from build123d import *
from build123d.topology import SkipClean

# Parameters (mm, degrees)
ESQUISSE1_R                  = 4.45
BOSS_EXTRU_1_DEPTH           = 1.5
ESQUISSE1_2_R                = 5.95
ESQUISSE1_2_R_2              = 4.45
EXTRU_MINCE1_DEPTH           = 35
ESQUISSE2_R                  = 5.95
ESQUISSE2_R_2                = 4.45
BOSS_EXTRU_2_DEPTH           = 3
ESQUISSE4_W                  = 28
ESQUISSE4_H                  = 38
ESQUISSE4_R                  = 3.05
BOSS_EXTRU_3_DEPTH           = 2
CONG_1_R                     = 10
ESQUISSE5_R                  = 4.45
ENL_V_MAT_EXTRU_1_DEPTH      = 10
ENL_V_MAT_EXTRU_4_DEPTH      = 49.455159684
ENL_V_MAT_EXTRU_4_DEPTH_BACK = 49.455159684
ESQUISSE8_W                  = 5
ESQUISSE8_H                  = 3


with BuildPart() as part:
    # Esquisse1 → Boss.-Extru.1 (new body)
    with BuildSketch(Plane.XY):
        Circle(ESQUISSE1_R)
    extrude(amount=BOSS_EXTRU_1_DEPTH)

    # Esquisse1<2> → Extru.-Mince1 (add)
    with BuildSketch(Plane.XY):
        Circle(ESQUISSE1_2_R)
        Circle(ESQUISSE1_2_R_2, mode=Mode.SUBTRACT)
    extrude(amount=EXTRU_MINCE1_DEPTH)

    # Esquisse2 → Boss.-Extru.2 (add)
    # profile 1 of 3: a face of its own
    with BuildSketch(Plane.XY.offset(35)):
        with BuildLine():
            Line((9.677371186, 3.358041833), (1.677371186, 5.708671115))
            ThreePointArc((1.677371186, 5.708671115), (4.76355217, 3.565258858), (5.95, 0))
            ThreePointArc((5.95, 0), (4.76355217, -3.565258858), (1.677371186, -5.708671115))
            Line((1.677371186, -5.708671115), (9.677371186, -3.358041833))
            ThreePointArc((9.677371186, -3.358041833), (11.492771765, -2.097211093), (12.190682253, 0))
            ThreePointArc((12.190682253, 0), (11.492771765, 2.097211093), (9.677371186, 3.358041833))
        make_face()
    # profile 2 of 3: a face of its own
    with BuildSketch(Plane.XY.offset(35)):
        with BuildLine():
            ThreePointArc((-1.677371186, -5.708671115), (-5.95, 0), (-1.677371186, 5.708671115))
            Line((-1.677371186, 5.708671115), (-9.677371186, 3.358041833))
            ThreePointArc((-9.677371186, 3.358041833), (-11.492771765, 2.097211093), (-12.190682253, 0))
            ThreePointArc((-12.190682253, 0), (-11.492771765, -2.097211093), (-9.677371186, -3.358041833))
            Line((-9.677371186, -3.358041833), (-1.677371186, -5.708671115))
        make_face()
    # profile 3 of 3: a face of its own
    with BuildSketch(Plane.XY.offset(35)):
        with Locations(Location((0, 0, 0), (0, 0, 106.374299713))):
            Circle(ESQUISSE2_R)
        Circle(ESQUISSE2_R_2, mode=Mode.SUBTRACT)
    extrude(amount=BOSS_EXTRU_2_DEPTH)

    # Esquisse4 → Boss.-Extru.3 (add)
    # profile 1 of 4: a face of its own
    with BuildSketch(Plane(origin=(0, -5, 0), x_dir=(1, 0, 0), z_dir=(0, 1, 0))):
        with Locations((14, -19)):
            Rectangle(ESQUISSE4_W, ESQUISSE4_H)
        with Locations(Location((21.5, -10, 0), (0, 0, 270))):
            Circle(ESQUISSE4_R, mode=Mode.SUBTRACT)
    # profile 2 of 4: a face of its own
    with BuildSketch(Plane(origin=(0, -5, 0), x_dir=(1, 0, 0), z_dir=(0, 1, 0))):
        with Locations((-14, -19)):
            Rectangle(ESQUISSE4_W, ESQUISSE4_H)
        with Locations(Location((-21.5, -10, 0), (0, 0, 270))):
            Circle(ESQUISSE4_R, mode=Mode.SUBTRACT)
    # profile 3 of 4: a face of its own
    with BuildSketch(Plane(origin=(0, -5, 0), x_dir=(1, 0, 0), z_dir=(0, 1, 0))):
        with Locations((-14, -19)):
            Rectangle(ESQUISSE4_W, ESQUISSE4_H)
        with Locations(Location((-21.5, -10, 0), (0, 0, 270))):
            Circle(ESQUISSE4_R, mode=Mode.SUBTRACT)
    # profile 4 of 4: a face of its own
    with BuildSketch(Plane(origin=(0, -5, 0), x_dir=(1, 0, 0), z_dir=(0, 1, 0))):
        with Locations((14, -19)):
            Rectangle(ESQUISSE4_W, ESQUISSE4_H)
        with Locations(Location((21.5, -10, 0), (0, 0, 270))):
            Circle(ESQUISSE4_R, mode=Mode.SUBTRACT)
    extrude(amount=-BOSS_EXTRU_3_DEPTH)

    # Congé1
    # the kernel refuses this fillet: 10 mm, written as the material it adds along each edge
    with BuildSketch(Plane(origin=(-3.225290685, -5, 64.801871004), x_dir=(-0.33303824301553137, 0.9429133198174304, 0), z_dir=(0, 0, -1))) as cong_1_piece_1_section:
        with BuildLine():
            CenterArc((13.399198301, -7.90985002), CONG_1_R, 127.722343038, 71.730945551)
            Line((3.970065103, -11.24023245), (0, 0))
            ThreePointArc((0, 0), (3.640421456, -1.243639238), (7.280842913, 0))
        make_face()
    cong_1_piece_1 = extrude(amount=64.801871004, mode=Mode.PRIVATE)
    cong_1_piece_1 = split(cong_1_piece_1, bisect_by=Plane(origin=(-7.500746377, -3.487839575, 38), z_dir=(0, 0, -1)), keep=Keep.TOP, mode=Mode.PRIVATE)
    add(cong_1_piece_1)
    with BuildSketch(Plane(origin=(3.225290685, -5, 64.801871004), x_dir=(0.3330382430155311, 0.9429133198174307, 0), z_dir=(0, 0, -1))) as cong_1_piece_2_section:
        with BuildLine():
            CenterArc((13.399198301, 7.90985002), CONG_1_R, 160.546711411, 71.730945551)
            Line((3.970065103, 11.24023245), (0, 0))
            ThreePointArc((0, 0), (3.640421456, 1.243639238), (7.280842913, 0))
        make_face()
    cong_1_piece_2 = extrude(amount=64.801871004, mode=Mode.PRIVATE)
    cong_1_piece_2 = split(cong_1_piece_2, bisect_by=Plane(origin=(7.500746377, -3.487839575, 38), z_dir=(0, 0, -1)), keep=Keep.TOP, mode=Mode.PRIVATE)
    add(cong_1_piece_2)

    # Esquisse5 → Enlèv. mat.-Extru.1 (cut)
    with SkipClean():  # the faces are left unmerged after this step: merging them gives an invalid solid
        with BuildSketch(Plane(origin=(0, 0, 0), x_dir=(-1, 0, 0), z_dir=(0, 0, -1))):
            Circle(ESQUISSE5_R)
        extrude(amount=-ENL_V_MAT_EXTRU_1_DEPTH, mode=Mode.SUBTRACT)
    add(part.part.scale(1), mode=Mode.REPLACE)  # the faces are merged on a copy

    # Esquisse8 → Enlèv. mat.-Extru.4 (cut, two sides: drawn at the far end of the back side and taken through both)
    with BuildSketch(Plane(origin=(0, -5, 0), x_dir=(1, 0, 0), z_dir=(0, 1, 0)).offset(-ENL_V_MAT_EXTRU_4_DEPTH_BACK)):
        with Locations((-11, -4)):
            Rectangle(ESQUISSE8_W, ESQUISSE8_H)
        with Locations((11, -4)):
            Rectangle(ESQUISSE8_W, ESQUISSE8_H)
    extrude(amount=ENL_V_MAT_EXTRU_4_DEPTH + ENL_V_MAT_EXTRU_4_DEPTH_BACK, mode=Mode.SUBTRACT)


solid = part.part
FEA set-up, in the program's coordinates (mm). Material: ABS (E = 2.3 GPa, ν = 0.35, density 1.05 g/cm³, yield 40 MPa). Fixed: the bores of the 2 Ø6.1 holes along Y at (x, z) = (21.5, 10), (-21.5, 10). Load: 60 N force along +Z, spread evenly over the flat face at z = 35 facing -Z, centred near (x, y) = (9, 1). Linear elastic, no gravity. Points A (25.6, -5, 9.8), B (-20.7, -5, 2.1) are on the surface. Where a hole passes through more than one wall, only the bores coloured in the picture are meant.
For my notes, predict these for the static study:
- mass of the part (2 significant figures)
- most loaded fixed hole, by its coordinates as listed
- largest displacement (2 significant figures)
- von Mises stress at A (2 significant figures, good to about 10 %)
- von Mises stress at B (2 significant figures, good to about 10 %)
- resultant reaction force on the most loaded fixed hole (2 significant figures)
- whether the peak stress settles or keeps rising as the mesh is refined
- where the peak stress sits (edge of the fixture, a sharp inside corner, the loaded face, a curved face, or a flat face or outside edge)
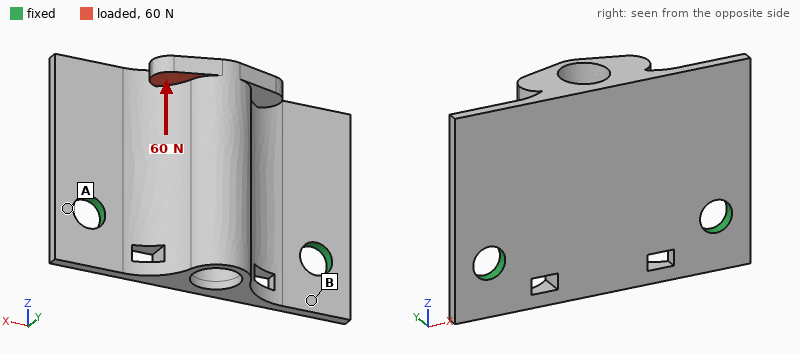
7.8 g
(21.5, 10)
0.62 mm
1.7 MPa
4.5 MPa
44 N
keeps rising
a sharp inside corner
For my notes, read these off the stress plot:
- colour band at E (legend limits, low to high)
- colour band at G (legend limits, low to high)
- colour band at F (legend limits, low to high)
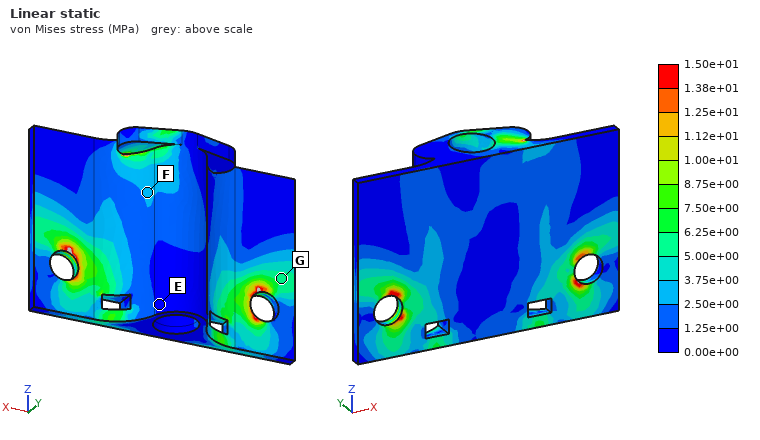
0.00e+00 to 1.25e+00 MPa
5.00e+00 to 6.25e+00 MPa
2.50e+00 to 3.75e+00 MPa
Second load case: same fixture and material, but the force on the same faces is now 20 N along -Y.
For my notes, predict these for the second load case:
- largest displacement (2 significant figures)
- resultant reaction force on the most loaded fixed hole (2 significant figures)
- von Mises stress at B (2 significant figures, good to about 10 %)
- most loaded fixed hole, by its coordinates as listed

0.70 mm
17 N
4.8 MPa
(21.5, 10)
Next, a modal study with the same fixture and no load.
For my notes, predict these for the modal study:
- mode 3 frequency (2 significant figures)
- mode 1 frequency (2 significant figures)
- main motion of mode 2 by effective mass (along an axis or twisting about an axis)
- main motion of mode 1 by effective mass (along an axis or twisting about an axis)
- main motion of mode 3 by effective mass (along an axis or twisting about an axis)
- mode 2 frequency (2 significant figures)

2100 Hz
570 Hz
twisting about Z
along Y
along Y
1800 Hz
